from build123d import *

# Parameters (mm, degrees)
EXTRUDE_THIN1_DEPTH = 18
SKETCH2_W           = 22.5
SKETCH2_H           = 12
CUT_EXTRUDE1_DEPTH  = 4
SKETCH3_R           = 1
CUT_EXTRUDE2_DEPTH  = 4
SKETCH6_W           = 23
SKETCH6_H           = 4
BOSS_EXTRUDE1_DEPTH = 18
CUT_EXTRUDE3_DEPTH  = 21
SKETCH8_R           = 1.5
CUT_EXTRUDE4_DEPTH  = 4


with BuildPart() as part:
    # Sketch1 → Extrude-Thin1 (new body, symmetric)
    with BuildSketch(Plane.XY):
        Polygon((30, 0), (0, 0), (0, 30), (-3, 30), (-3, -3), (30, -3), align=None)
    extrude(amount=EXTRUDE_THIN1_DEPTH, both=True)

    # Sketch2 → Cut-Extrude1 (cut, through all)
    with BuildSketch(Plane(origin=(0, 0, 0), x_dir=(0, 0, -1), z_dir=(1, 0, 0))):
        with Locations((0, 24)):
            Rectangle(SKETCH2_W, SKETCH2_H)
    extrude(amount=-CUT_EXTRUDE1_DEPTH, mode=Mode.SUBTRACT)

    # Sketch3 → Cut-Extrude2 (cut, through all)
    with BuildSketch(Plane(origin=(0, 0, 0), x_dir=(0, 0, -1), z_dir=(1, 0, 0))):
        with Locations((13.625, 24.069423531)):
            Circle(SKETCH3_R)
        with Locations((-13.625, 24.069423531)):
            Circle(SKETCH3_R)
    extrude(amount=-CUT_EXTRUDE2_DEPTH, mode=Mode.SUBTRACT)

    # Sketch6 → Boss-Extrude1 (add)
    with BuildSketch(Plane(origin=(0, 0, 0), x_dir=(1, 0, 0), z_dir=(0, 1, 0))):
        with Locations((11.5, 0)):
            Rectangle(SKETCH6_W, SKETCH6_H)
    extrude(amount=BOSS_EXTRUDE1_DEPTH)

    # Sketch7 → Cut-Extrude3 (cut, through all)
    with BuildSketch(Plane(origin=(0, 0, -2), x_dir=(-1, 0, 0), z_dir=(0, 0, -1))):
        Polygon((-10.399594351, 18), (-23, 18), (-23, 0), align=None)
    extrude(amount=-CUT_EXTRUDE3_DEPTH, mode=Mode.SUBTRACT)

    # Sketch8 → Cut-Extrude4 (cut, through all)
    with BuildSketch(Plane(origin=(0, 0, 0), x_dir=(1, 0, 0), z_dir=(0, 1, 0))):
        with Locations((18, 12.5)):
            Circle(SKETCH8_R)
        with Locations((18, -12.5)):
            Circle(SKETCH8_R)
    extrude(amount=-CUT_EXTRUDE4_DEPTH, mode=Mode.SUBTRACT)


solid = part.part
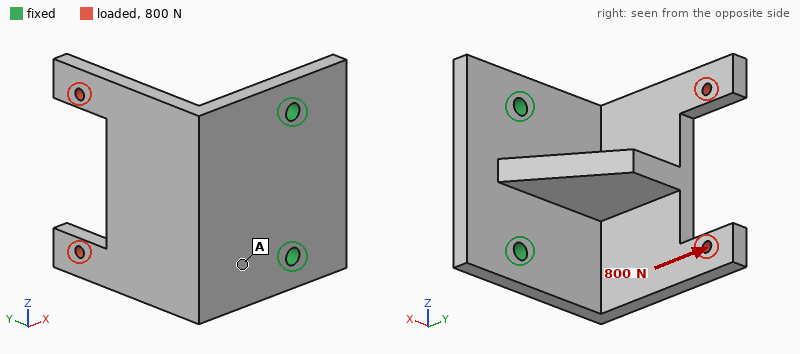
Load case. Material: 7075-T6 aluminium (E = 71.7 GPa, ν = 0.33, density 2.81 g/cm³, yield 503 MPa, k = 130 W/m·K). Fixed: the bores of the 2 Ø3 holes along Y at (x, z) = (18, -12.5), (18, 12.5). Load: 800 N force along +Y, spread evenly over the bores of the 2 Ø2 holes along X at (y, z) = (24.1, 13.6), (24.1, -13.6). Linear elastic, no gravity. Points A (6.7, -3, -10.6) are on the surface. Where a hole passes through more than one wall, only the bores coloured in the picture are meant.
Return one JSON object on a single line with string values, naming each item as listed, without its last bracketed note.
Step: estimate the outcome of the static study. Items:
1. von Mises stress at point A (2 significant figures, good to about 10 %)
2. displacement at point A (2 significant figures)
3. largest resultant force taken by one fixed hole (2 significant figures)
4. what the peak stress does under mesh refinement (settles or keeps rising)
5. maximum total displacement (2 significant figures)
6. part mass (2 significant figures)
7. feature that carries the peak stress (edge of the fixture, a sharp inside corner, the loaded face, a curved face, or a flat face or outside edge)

{"von Mises stress at point A": "45 MPa", "displacement at point A": "0.12 mm", "largest resultant force taken by one fixed hole": "420 N", "what the peak stress does under mesh refinement": "keeps rising", "maximum total displacement": "0.48 mm", "part mass": "20 g", "feature that carries the peak stress": "edge of the fixture"}
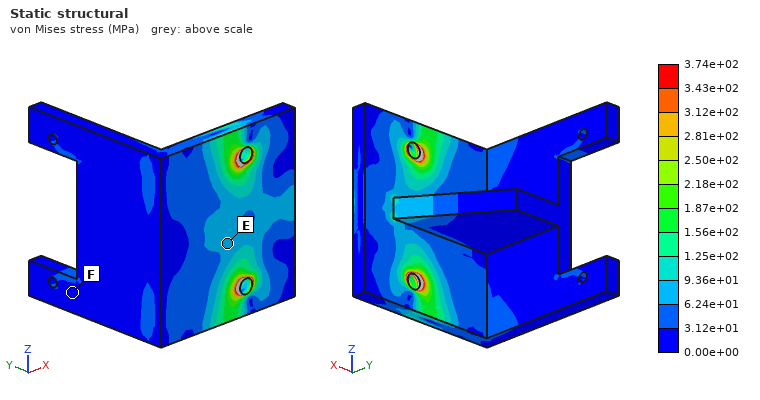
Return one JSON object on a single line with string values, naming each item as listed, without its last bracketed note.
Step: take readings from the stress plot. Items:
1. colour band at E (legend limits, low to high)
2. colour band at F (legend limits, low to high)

{"colour band at E": "6.24e+01 to 9.36e+01 MPa", "colour band at F": "0.00e+00 to 3.12e+01 MPa"}
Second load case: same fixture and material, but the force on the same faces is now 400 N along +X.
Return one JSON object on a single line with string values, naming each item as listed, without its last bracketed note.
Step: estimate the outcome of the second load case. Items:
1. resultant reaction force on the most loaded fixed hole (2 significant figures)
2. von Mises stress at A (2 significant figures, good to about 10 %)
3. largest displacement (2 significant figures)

{"resultant reaction force on the most loaded fixed hole": "210 N", "von Mises stress at A": "32 MPa", "largest displacement": "0.63 mm"}
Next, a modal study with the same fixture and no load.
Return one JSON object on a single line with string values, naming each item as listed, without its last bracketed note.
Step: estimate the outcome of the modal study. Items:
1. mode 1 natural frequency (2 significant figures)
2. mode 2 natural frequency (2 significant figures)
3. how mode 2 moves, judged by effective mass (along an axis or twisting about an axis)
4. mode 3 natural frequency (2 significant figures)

{"mode 1 natural frequency": "2300 Hz", "mode 2 natural frequency": "3600 Hz", "how mode 2 moves, judged by effective mass": "along Z", "mode 3 natural frequency": "4900 Hz"}
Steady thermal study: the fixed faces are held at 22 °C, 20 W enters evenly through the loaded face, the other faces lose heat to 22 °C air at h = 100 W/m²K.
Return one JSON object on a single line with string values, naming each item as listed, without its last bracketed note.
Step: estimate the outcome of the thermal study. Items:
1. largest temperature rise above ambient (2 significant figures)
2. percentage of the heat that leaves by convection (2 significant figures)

{"largest temperature rise above ambient": "66 K", "percentage of the heat that leaves by convection": "43 %"}
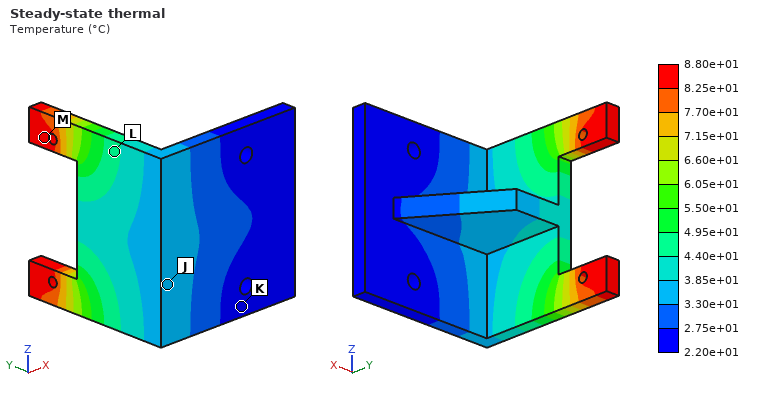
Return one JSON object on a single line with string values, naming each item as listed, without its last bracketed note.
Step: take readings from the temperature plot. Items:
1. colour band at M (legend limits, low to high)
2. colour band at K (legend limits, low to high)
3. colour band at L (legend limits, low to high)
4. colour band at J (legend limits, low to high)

{"colour band at M": "8.25e+01 to 8.80e+01 °C", "colour band at K": "2.20e+01 to 2.75e+01 °C", "colour band at L": "4.40e+01 to 4.95e+01 °C", "colour band at J": "3.30e+01 to 3.85e+01 °C"}
